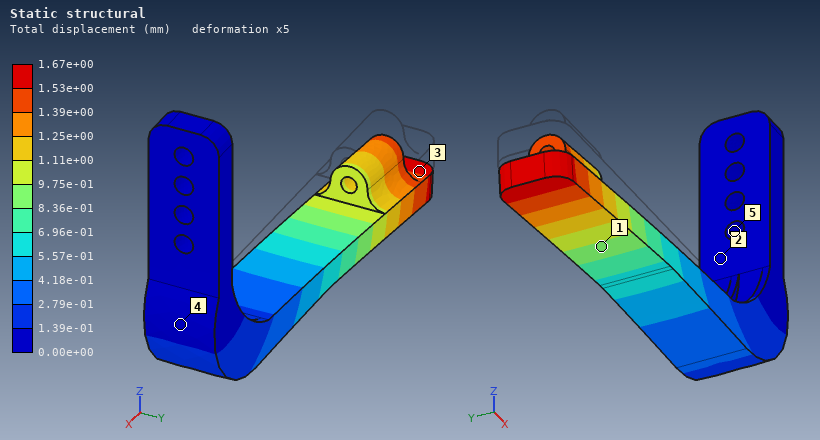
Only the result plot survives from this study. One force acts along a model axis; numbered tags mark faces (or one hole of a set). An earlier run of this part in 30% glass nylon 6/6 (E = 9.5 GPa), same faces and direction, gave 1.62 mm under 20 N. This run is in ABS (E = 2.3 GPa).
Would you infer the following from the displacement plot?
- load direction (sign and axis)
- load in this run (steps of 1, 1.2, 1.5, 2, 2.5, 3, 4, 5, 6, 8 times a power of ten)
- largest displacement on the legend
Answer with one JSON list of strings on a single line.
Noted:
["-Z", "5 N", "1.67e+00 mm"]
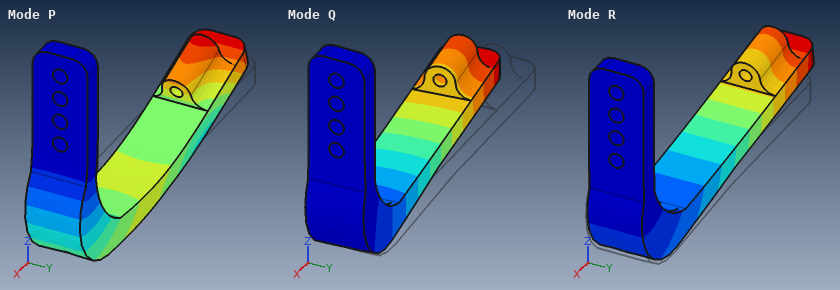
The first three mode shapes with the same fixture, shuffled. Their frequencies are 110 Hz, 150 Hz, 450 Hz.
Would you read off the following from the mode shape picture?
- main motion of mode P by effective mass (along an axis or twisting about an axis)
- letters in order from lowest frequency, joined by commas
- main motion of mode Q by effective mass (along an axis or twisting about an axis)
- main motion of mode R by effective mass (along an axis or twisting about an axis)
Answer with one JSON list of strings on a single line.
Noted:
["along X", "R, Q, P", "along Y", "along Z"]
